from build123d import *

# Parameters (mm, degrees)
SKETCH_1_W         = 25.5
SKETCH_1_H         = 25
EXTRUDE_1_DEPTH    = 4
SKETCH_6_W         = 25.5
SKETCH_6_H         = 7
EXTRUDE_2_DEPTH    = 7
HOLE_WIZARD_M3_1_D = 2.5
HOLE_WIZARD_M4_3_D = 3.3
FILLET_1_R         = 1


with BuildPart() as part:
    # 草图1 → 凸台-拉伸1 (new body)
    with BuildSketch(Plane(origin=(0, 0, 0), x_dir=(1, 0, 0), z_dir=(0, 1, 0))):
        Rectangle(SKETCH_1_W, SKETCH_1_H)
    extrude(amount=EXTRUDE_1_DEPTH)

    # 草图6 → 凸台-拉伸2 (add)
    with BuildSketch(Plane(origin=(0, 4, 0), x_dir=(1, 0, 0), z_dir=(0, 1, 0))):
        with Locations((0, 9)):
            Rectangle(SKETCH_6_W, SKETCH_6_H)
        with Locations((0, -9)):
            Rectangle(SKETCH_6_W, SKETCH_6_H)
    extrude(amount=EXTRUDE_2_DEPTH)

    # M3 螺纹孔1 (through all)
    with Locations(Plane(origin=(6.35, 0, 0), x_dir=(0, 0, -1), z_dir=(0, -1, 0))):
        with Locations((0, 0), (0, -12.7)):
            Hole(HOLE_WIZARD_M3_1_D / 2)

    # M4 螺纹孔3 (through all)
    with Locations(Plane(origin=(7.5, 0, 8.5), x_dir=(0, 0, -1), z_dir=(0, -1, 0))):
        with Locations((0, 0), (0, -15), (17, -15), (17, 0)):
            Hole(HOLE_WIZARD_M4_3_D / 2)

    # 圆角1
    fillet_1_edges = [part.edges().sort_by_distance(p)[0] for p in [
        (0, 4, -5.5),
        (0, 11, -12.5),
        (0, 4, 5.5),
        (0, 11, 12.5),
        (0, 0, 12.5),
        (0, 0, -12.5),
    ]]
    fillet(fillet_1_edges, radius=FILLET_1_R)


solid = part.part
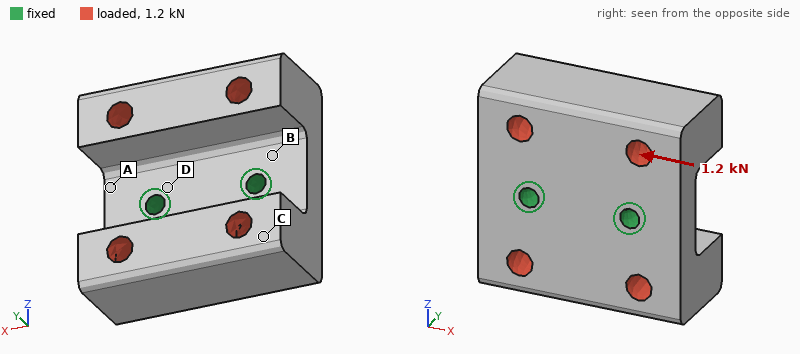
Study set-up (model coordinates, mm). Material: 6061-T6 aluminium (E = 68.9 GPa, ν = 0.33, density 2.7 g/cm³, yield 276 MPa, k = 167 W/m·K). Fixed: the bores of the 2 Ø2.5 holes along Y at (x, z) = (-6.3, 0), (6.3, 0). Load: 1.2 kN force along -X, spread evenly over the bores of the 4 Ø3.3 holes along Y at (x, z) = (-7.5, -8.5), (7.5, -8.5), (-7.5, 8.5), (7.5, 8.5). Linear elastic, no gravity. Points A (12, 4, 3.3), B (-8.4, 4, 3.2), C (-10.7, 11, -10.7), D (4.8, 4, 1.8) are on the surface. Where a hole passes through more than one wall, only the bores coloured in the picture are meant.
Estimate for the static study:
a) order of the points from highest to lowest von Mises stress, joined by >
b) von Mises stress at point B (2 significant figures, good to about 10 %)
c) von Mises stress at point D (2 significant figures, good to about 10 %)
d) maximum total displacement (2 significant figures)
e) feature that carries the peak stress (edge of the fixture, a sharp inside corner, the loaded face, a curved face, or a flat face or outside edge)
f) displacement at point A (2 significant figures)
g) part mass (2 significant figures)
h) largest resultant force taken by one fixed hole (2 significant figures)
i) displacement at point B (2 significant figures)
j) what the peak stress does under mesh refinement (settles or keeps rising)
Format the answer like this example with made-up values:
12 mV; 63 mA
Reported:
D > B > A > C; 16 MPa; 22 MPa; 7.0 µm; edge of the fixture; 2.8 µm; 12 g; 650 N; 1.8 µm; keeps rising
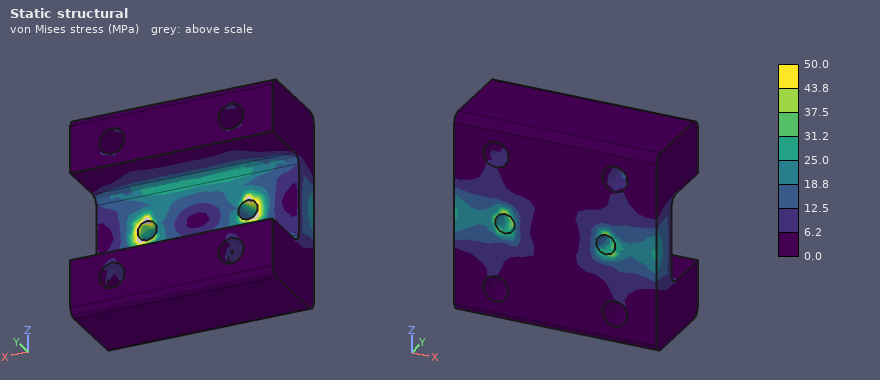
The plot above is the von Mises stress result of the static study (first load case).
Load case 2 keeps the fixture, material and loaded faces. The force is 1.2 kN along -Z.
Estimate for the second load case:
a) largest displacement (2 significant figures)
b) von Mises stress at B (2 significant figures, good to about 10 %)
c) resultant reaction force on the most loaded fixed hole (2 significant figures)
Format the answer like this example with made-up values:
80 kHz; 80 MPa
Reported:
25 µm; 39 MPa; 600 N
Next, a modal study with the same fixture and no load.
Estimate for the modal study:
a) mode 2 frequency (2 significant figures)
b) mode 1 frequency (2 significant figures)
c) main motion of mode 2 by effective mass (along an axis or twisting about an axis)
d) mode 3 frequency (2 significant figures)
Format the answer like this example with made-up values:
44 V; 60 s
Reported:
11 kHz; 9100 Hz; along Y; 18 kHz
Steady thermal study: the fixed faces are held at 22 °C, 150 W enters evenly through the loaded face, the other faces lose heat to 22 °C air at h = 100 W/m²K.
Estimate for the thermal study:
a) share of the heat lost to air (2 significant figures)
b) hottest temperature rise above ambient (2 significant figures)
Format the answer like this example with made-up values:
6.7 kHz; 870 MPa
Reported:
6.0 %; 50 K
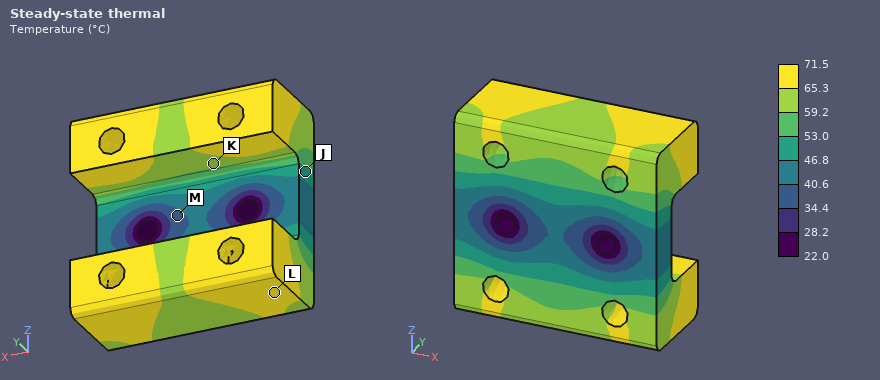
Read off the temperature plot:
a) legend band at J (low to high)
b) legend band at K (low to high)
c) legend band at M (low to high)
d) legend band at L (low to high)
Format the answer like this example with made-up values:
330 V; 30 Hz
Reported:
46.8 to 53.0 °C; 59.2 to 65.3 °C; 34.4 to 40.6 °C; 65.3 to 71.5 °C
